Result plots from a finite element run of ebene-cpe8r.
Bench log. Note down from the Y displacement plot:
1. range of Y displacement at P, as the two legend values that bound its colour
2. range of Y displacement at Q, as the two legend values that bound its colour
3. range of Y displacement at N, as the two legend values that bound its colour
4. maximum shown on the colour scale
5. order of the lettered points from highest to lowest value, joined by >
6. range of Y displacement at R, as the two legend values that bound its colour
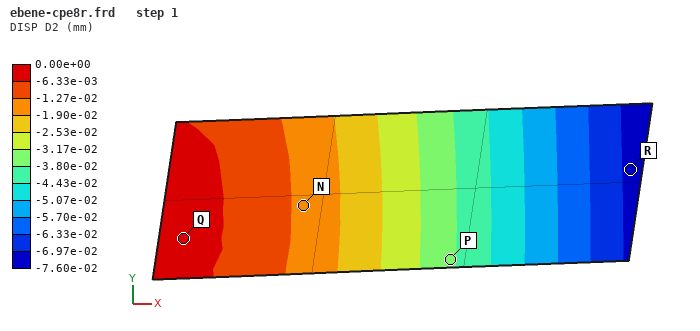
-3.80e-02 to -3.17e-02 mm
-6.33e-03 to 0.00e+00 mm
-1.90e-02 to -1.27e-02 mm
0.00e+00 mm
Q > N > P > R
-7.60e-02 to -6.97e-02 mm
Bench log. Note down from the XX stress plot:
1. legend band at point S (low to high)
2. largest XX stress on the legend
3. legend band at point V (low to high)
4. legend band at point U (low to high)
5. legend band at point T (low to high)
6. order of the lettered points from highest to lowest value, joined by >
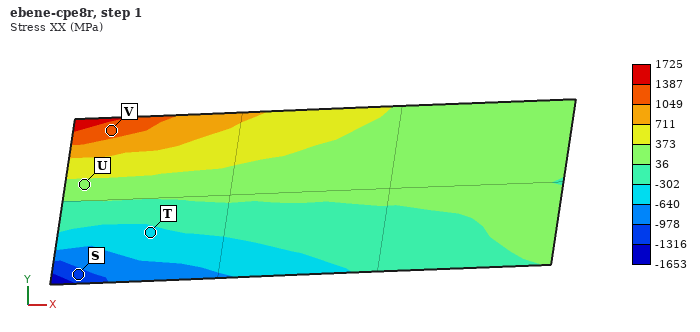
-1316 to -978 MPa
1725 MPa
1049 to 1387 MPa
36 to 373 MPa
-640 to -302 MPa
V > U > T > S
